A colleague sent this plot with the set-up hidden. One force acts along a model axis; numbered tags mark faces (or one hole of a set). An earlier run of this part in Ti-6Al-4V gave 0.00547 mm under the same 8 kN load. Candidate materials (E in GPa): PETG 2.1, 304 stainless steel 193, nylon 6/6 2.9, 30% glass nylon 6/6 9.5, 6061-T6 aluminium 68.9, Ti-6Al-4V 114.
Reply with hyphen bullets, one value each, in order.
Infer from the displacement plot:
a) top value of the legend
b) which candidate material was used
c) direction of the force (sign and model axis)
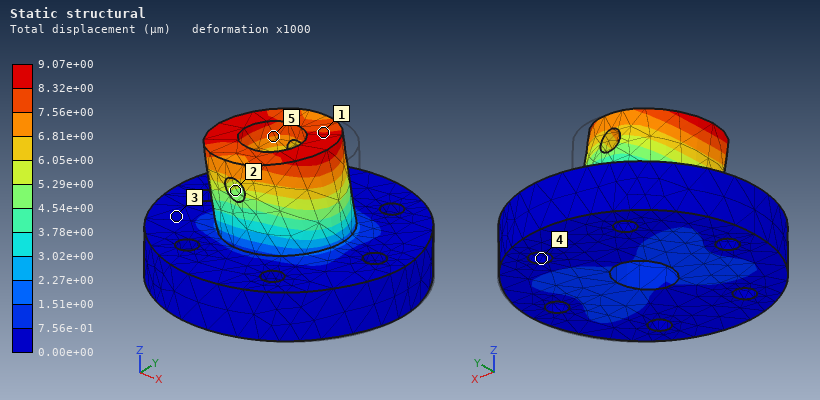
- 9.07e+00 µm
- 6061-T6 aluminium
- -X
